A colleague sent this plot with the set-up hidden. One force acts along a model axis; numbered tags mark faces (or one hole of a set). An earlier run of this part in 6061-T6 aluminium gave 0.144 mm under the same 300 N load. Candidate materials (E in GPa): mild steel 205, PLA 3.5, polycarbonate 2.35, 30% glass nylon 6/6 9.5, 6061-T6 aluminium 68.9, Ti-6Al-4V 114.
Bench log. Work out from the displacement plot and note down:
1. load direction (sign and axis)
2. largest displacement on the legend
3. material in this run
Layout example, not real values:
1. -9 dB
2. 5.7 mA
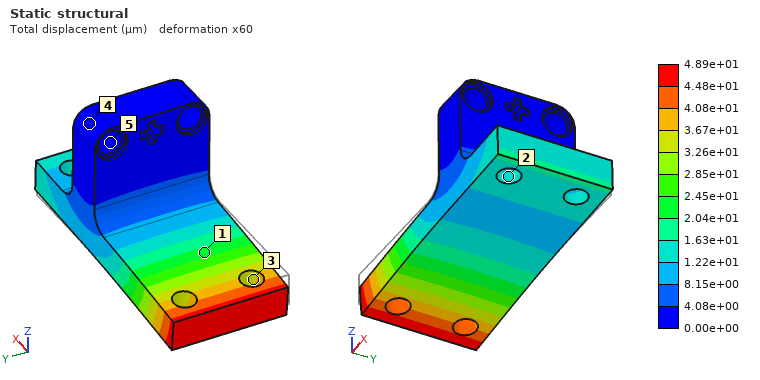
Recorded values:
1. -Z
2. 4.89e+01 µm
3. mild steel
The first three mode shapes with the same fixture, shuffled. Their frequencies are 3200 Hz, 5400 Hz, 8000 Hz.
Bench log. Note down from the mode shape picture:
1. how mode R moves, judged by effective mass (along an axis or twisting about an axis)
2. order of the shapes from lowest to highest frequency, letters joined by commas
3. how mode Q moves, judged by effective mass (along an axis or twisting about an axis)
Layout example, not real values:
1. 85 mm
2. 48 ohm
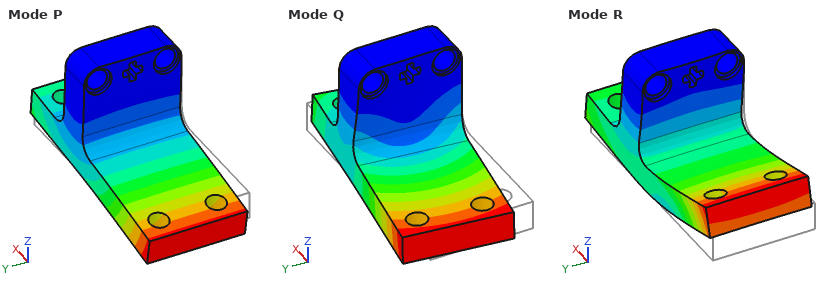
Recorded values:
1. along X
2. P, Q, R
3. along Y
